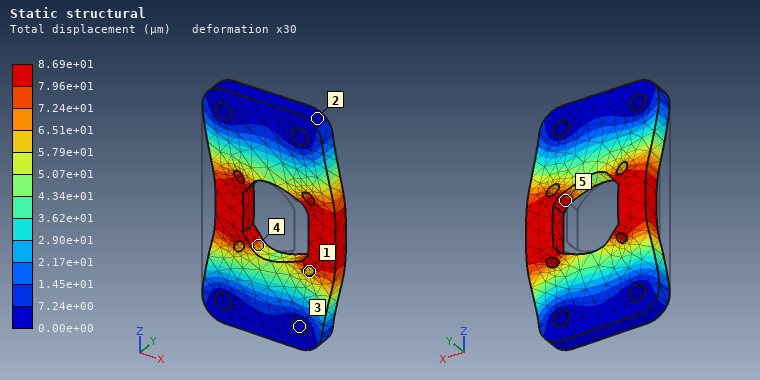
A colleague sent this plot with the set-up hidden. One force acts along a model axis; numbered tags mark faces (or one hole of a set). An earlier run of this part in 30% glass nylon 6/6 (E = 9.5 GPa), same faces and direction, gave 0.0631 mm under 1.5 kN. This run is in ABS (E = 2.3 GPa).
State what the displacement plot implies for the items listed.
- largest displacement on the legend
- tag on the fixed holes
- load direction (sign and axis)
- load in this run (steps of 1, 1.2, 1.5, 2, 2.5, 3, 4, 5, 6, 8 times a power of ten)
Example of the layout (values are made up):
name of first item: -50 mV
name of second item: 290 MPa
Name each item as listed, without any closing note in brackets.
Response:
largest displacement on the legend: 8.69e+01 µm
tag on the fixed holes: 3
load direction: +X
load in this run: 500 N
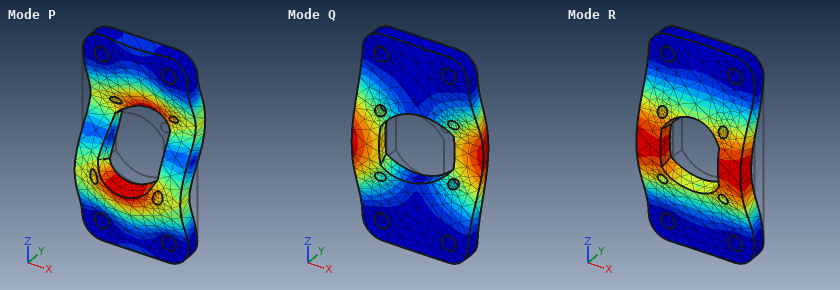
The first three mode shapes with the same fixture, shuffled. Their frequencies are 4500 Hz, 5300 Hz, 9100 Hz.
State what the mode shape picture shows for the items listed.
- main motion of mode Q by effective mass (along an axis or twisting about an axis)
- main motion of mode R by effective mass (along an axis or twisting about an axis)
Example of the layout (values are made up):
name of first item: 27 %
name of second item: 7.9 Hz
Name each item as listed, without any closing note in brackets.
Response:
main motion of mode Q by effective mass: twisting about Z
main motion of mode R by effective mass: along Y
